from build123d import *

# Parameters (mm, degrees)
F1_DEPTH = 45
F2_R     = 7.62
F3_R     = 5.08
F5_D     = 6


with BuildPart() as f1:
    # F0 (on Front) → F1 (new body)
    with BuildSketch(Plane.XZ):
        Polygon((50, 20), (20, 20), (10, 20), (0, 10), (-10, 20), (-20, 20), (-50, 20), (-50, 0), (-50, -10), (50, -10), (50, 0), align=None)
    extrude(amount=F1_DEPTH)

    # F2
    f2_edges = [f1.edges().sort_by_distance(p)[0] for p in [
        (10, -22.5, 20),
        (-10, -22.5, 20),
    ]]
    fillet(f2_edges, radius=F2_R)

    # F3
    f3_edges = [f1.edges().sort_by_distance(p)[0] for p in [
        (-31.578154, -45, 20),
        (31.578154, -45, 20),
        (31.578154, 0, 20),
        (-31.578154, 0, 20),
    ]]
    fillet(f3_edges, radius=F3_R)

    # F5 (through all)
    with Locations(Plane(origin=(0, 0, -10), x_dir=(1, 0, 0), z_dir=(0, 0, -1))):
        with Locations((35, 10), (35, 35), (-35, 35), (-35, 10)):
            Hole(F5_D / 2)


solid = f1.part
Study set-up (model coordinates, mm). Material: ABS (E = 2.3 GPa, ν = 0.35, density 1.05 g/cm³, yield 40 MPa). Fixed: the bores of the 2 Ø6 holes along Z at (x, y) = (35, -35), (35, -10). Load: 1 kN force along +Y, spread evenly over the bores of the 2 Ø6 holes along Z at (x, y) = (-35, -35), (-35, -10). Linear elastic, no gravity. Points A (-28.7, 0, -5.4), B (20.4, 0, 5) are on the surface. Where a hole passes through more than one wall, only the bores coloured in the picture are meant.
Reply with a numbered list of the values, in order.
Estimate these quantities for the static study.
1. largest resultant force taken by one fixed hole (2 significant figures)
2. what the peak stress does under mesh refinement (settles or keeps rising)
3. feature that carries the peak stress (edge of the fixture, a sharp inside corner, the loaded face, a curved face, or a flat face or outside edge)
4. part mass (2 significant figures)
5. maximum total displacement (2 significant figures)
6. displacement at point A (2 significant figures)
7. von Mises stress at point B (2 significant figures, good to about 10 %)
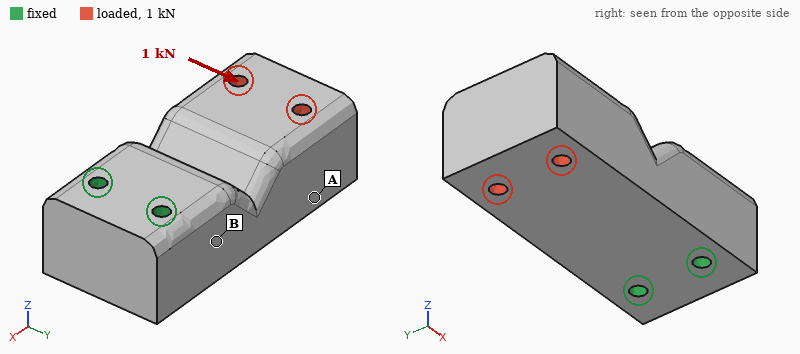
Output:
1. 2.5 kN
2. keeps rising
3. edge of the fixture
4. 130 g
5. 0.48 mm
6. 0.34 mm
7. 5.5 MPa
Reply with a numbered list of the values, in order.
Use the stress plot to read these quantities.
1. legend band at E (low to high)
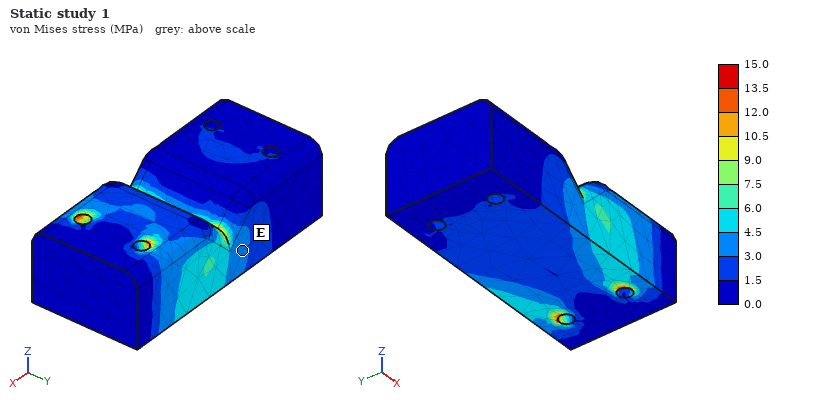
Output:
1. 3.0 to 4.5 MPa
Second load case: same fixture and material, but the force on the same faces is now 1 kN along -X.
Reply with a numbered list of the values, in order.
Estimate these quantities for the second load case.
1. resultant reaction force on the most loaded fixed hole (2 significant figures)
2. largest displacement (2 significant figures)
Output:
1. 510 N
2. 71 µm
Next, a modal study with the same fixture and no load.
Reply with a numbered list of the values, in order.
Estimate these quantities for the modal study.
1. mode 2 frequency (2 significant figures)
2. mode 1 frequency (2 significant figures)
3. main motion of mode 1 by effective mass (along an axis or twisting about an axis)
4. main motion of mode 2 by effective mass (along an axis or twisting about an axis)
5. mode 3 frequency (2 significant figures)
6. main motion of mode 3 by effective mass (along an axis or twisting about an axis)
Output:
1. 1100 Hz
2. 800 Hz
3. along Z
4. along Y
5. 2200 Hz
6. twisting about X
